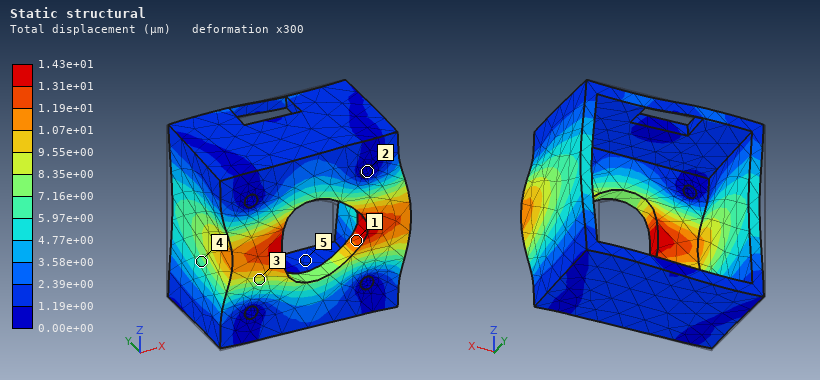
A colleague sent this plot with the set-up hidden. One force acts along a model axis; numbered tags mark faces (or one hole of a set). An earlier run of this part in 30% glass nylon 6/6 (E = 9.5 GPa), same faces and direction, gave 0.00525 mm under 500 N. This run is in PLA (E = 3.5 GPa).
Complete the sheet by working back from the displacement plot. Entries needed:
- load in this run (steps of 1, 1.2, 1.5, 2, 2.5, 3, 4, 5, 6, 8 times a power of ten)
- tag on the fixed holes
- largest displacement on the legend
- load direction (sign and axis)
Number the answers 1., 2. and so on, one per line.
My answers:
1. 500 N
2. 2
3. 1.43e+01 µm
4. +X
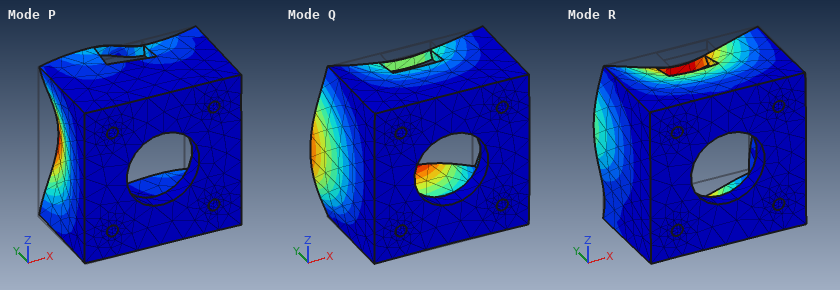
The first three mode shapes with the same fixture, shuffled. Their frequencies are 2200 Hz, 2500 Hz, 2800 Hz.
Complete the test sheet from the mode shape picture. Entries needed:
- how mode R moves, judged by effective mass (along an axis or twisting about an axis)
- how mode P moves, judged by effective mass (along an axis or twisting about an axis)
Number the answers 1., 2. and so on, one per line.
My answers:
1. along Z
2. along X
